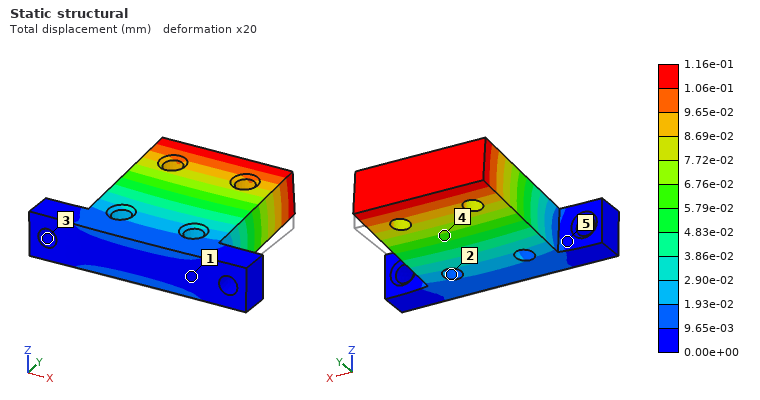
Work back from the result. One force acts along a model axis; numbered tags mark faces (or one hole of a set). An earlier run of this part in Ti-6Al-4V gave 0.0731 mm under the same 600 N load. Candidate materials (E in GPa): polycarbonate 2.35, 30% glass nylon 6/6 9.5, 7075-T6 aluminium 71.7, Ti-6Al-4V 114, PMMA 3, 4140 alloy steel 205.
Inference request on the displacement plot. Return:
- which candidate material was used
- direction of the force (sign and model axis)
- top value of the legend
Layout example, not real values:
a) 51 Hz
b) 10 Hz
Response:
a) 7075-T6 aluminium
b) +Z
c) 1.16e-01 mm
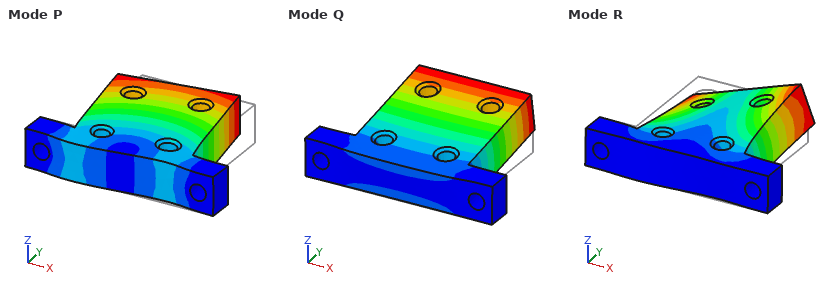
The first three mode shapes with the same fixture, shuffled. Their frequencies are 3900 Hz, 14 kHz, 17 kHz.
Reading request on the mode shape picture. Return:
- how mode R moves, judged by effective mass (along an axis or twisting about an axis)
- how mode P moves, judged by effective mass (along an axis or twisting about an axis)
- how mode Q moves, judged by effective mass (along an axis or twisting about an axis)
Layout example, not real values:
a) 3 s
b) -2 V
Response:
a) twisting about Y
b) along X
c) along Z
